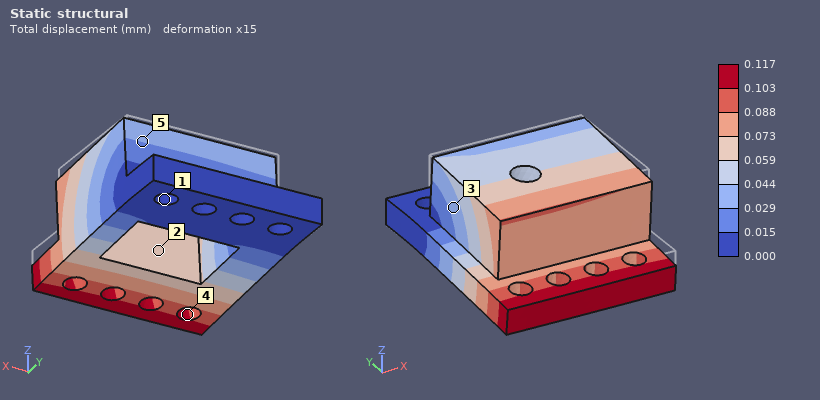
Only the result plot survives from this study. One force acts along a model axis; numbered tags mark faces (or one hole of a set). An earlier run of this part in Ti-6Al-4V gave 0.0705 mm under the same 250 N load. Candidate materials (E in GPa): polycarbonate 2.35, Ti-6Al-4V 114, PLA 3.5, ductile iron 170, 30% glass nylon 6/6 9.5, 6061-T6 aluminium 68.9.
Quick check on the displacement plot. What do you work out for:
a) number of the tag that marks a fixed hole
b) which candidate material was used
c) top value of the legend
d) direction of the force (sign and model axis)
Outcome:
1
6061-T6 aluminium
0.117 mm
-Z
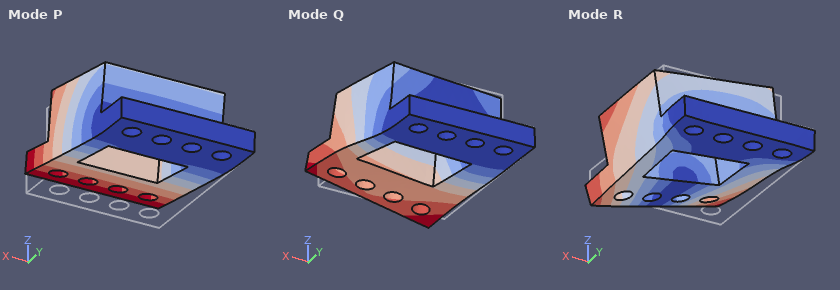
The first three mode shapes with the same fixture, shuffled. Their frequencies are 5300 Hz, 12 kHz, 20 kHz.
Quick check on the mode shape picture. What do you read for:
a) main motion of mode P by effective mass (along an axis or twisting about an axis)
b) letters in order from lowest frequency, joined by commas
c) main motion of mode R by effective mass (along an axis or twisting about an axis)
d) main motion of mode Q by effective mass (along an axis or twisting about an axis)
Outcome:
along Z
P, Q, R
along X
along X
